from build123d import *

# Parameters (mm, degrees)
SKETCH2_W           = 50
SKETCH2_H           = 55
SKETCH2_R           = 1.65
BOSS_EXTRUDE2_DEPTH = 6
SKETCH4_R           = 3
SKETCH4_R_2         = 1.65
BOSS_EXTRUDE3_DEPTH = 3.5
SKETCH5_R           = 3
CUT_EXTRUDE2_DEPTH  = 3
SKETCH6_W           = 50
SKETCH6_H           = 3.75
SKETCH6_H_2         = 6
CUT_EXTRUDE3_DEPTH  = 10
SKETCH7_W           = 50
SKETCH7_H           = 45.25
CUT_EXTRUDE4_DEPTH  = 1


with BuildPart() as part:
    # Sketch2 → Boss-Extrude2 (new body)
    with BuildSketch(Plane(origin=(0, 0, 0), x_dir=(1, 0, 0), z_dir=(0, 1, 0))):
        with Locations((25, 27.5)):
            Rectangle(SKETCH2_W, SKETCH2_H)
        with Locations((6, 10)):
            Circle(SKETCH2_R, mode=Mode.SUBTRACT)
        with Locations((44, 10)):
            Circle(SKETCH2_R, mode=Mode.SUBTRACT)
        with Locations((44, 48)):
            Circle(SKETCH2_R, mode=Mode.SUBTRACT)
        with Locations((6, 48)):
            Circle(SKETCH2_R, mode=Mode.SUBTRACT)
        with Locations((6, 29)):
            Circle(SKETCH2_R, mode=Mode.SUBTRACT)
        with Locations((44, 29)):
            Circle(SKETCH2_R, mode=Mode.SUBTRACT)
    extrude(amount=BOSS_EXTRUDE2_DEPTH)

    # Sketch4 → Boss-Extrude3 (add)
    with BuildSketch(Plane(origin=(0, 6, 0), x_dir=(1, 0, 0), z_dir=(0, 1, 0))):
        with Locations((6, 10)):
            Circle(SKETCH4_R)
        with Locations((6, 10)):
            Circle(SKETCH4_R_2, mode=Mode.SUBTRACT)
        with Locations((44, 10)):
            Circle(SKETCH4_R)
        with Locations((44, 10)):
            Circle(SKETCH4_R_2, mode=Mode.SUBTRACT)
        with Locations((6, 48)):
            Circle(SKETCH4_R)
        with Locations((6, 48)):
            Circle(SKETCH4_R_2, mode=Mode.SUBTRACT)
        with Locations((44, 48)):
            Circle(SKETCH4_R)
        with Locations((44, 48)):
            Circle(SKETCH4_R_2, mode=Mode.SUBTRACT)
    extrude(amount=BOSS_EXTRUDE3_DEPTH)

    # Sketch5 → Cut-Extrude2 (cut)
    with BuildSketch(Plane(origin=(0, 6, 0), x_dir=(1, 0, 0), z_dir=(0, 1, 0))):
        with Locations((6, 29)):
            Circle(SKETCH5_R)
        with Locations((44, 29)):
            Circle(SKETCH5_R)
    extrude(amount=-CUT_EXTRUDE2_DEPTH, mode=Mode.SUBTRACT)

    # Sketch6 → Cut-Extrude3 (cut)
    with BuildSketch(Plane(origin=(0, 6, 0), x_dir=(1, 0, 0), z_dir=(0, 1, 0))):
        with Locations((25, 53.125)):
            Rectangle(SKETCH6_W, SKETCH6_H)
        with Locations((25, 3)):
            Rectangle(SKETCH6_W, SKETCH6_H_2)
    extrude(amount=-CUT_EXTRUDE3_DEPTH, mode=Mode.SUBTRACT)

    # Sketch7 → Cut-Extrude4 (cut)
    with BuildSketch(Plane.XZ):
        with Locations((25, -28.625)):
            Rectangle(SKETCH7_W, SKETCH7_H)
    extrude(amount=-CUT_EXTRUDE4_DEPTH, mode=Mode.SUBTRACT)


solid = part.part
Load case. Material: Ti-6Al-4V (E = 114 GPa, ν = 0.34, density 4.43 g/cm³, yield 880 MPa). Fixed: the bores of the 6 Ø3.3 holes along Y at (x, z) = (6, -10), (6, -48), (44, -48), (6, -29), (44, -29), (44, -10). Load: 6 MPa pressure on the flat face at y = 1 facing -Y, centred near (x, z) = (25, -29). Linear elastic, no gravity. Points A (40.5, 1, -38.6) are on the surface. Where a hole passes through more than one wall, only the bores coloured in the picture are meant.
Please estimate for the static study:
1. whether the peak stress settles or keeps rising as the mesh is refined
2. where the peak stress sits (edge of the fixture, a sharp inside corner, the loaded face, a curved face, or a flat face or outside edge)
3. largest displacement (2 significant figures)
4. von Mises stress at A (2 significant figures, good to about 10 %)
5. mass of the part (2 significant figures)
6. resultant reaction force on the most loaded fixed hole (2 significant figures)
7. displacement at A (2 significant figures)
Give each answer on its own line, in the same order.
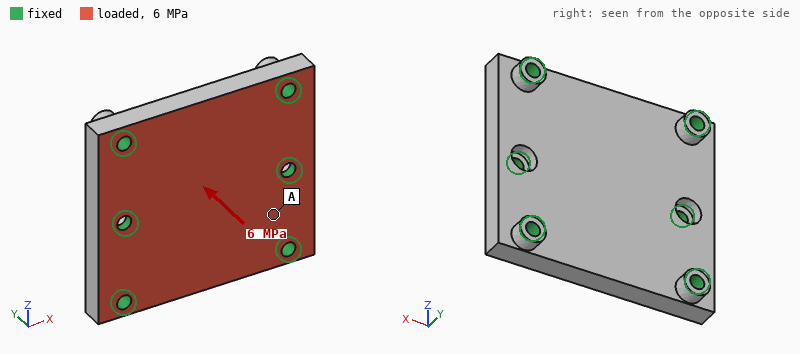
keeps rising
edge of the fixture
43 µm
47 MPa
50 g
2.6 kN
14 µm
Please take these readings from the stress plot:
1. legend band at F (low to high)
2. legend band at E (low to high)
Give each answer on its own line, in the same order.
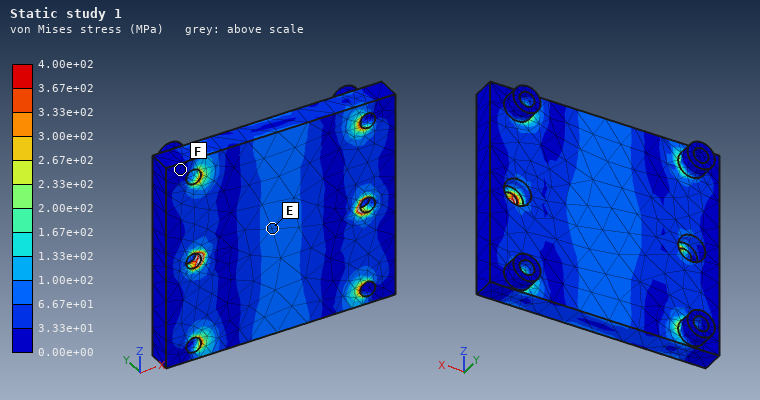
0.00e+00 to 3.33e+01 MPa
6.67e+01 to 1.00e+02 MPa
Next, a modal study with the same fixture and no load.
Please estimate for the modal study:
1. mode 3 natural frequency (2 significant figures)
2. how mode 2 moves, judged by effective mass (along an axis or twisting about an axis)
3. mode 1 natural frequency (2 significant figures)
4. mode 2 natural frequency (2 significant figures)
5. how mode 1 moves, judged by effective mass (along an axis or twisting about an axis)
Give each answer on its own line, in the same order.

26 kHz
twisting about X
15 kHz
19 kHz
along Y
